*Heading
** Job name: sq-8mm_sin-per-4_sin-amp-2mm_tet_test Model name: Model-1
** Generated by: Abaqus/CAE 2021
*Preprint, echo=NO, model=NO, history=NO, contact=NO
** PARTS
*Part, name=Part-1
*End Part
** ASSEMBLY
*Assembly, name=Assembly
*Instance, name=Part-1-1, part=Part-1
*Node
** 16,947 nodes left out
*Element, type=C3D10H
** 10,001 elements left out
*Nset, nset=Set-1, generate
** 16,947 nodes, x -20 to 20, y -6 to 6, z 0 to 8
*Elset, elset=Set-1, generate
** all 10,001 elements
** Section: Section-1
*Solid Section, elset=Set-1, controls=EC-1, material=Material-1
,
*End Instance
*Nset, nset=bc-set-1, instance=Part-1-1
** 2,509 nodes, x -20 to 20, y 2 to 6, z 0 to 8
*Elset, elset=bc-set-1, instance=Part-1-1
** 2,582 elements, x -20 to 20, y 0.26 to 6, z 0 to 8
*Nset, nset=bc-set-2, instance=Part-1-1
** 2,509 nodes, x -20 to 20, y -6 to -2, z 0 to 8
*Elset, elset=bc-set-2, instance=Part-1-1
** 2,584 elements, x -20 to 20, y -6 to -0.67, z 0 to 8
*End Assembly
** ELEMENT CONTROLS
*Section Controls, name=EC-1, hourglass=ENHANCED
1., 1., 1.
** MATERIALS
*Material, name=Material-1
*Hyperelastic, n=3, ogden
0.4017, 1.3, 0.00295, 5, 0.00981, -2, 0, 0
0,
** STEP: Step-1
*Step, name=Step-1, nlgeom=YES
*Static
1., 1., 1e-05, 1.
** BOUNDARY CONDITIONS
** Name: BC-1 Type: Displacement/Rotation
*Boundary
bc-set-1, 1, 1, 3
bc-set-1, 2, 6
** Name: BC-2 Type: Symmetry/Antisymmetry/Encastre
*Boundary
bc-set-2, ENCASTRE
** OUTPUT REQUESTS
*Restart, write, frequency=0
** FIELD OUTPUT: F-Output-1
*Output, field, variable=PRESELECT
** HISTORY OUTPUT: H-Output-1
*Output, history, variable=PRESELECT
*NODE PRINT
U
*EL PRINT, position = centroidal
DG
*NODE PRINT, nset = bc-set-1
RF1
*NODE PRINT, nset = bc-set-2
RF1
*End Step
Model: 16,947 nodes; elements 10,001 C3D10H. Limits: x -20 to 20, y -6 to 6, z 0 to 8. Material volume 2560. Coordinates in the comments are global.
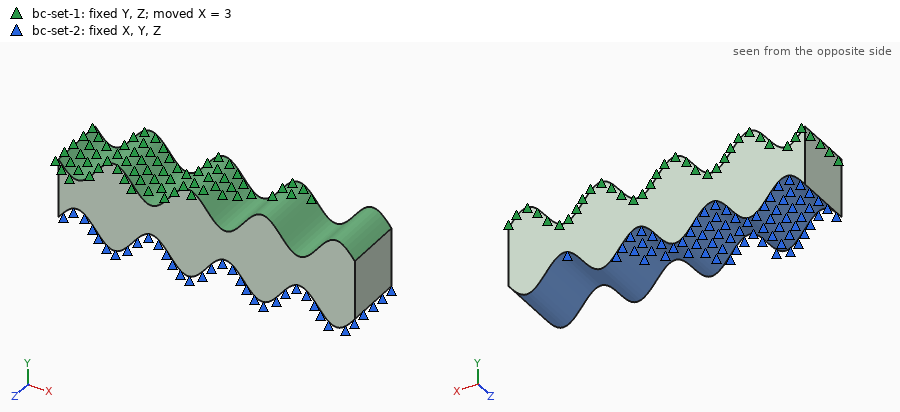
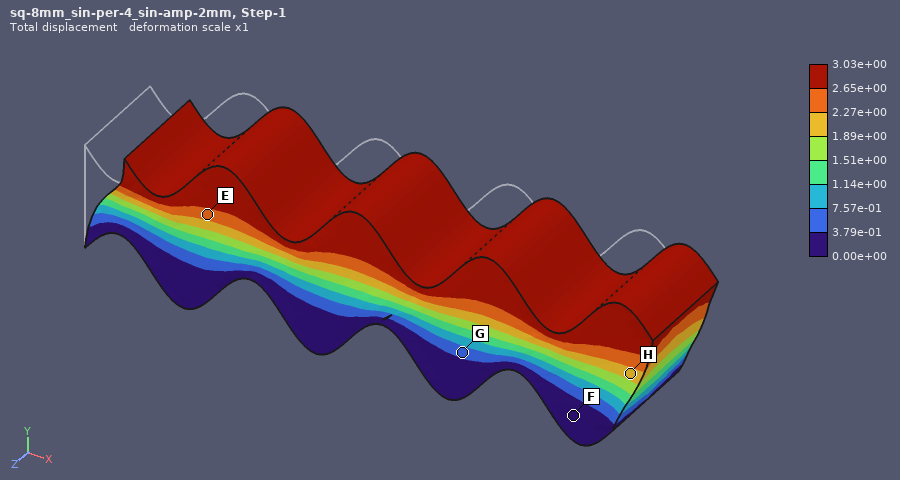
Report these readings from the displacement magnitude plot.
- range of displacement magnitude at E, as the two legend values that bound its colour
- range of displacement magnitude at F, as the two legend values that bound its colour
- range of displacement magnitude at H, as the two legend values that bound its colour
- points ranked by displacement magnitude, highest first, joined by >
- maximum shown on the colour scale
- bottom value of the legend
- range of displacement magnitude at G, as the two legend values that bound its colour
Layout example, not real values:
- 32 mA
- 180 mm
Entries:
- 2.27e+00 to 2.65e+00
- 0.00e+00 to 3.79e-01
- 1.89e+00 to 2.27e+00
- E > H > G > F
- 3.03e+00
- 0.00e+00
- 3.79e-01 to 7.57e-01
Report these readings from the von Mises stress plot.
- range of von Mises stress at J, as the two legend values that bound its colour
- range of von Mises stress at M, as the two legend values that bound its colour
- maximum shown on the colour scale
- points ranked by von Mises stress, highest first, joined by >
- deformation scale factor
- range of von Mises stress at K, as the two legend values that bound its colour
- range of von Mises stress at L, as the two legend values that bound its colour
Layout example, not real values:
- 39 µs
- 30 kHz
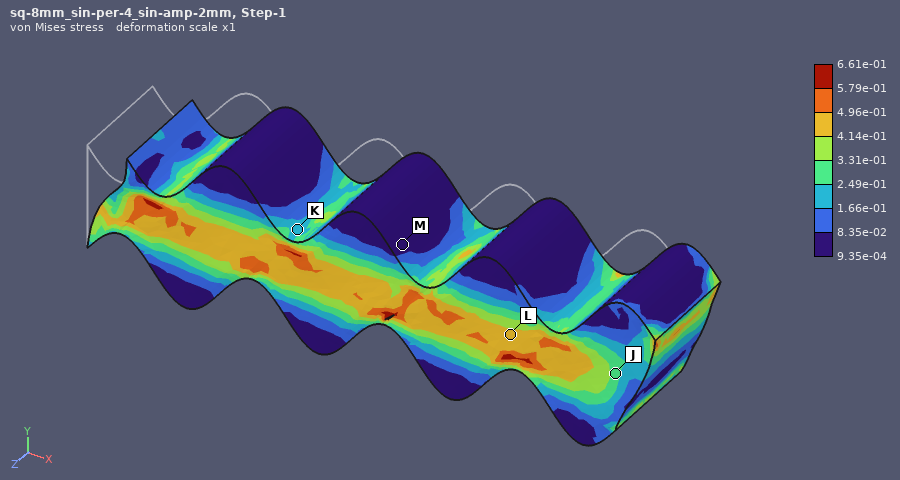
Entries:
- 2.49e-01 to 3.31e-01
- 9.35e-04 to 8.35e-02
- 6.61e-01
- L > J > K > M
- 1
- 1.66e-01 to 2.49e-01
- 4.14e-01 to 4.96e-01
